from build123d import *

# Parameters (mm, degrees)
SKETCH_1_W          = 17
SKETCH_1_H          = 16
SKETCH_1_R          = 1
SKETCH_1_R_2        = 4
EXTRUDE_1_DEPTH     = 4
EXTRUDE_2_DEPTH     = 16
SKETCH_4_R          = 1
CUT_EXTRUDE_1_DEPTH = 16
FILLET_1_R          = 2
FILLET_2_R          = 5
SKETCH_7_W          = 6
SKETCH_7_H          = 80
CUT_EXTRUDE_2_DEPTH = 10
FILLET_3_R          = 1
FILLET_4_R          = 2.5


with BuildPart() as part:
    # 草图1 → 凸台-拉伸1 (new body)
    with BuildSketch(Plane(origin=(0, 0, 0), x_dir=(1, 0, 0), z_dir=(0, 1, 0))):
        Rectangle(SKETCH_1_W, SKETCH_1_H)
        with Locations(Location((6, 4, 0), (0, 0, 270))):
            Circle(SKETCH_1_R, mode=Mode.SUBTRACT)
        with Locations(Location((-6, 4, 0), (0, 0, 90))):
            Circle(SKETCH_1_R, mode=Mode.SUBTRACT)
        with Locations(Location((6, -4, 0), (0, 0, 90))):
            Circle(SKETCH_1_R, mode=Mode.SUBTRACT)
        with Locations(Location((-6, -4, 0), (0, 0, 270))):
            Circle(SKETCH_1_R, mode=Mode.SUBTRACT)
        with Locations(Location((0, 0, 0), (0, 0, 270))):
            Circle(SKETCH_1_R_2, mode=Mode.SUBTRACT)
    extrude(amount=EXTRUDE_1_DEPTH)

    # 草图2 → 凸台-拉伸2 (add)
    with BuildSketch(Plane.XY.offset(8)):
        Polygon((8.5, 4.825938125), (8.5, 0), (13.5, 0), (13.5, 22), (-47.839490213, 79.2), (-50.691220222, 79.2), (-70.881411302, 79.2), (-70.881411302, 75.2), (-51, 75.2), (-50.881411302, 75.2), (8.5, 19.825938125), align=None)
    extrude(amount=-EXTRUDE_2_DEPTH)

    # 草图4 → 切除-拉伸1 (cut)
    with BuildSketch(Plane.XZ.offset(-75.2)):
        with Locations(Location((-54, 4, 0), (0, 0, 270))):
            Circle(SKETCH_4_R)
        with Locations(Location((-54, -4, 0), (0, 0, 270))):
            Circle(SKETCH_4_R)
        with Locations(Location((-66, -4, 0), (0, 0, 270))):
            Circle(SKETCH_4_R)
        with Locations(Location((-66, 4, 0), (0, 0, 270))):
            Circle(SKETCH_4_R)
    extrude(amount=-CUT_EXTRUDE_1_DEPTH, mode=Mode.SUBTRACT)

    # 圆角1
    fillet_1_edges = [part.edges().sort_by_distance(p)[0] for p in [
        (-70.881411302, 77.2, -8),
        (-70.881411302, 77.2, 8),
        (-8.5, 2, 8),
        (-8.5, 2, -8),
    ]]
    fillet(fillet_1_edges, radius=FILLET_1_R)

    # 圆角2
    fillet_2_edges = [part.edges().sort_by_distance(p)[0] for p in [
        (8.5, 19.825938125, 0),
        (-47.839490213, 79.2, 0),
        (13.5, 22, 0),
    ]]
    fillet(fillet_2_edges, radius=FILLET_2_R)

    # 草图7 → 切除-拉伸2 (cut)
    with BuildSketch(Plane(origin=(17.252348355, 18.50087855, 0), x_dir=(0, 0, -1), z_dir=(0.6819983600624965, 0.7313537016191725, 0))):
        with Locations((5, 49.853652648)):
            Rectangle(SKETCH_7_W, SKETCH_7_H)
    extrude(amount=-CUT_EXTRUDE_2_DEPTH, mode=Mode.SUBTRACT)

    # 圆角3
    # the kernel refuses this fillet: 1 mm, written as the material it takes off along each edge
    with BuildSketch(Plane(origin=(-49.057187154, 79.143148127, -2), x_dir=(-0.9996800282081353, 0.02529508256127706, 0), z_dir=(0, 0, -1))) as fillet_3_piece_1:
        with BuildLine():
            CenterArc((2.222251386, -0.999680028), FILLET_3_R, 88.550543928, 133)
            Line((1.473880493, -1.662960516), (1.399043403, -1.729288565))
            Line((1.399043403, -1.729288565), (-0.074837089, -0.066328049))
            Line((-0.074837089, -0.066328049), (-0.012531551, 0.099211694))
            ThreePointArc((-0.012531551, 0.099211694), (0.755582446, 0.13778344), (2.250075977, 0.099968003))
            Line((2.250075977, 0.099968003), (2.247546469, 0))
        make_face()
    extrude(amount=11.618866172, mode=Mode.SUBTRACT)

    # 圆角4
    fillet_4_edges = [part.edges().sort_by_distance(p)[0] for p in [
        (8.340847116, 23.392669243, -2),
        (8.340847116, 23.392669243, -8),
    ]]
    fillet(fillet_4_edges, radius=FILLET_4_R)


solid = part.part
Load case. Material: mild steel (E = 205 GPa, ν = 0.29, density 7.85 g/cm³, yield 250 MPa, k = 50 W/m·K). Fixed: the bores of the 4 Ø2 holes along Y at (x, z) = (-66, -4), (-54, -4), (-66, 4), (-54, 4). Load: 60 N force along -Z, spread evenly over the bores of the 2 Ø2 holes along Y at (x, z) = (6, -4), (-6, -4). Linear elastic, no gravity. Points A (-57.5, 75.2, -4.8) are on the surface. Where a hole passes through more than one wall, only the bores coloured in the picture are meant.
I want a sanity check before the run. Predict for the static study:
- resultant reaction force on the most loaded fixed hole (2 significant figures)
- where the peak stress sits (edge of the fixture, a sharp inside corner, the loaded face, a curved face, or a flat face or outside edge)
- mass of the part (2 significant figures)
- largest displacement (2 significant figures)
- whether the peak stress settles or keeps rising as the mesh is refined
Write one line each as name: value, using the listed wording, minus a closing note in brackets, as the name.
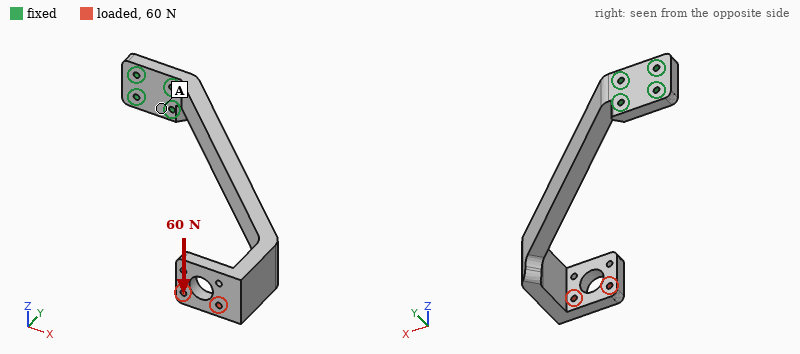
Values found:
resultant reaction force on the most loaded fixed hole: 520 N
where the peak stress sits: edge of the fixture
mass of the part: 63 g
largest displacement: 0.36 mm
whether the peak stress settles or keeps rising as the mesh is refined: keeps rising
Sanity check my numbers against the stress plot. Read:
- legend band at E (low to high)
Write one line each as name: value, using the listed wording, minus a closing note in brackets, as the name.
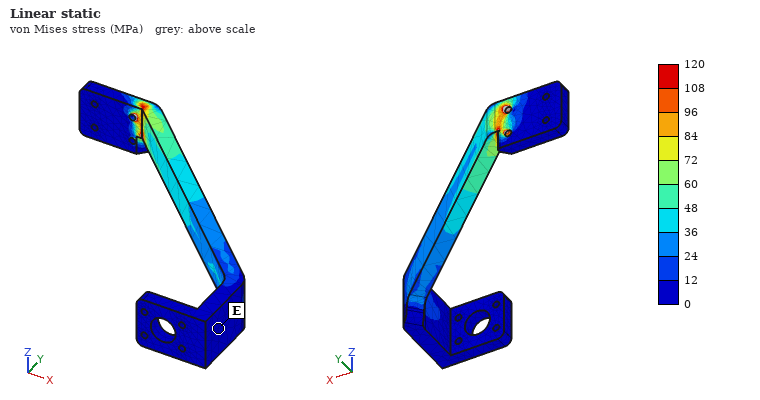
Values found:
legend band at E: 0 to 12 MPa
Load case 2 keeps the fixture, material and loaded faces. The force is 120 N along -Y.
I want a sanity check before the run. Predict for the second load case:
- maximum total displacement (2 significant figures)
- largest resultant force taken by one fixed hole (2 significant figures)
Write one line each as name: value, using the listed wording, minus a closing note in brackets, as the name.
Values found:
maximum total displacement: 0.98 mm
largest resultant force taken by one fixed hole: 130 N
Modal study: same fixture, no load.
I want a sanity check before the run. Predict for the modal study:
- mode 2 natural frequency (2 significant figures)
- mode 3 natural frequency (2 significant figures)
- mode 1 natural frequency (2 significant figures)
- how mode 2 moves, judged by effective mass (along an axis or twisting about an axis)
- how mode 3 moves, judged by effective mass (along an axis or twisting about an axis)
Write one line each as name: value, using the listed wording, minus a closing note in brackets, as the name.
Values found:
mode 2 natural frequency: 470 Hz
mode 3 natural frequency: 1600 Hz
mode 1 natural frequency: 250 Hz
how mode 2 moves, judged by effective mass: along Z
how mode 3 moves, judged by effective mass: along Y
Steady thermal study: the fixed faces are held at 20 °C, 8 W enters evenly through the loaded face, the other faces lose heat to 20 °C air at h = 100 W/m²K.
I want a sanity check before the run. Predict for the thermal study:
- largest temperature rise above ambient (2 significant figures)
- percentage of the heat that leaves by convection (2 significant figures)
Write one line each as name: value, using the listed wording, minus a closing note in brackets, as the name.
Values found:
largest temperature rise above ambient: 63 K
percentage of the heat that leaves by convection: 98 %
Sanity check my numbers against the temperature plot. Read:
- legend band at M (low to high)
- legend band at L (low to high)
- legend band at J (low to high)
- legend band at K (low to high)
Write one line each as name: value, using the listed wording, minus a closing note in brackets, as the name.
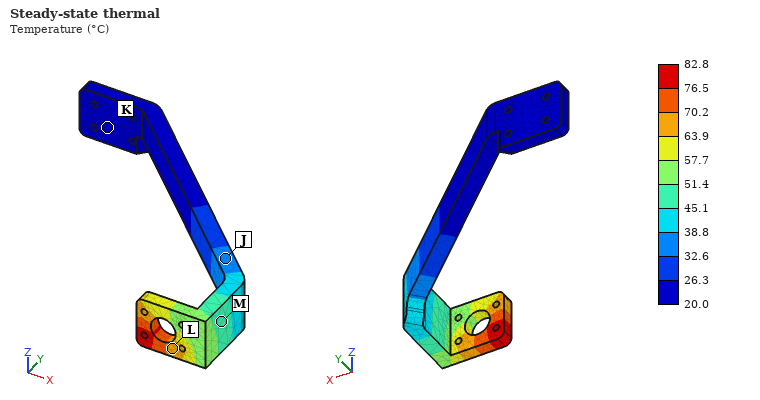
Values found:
legend band at M: 45.1 to 51.4 °C
legend band at L: 63.9 to 70.2 °C
legend band at J: 32.6 to 38.8 °C
legend band at K: 20.0 to 26.3 °C
